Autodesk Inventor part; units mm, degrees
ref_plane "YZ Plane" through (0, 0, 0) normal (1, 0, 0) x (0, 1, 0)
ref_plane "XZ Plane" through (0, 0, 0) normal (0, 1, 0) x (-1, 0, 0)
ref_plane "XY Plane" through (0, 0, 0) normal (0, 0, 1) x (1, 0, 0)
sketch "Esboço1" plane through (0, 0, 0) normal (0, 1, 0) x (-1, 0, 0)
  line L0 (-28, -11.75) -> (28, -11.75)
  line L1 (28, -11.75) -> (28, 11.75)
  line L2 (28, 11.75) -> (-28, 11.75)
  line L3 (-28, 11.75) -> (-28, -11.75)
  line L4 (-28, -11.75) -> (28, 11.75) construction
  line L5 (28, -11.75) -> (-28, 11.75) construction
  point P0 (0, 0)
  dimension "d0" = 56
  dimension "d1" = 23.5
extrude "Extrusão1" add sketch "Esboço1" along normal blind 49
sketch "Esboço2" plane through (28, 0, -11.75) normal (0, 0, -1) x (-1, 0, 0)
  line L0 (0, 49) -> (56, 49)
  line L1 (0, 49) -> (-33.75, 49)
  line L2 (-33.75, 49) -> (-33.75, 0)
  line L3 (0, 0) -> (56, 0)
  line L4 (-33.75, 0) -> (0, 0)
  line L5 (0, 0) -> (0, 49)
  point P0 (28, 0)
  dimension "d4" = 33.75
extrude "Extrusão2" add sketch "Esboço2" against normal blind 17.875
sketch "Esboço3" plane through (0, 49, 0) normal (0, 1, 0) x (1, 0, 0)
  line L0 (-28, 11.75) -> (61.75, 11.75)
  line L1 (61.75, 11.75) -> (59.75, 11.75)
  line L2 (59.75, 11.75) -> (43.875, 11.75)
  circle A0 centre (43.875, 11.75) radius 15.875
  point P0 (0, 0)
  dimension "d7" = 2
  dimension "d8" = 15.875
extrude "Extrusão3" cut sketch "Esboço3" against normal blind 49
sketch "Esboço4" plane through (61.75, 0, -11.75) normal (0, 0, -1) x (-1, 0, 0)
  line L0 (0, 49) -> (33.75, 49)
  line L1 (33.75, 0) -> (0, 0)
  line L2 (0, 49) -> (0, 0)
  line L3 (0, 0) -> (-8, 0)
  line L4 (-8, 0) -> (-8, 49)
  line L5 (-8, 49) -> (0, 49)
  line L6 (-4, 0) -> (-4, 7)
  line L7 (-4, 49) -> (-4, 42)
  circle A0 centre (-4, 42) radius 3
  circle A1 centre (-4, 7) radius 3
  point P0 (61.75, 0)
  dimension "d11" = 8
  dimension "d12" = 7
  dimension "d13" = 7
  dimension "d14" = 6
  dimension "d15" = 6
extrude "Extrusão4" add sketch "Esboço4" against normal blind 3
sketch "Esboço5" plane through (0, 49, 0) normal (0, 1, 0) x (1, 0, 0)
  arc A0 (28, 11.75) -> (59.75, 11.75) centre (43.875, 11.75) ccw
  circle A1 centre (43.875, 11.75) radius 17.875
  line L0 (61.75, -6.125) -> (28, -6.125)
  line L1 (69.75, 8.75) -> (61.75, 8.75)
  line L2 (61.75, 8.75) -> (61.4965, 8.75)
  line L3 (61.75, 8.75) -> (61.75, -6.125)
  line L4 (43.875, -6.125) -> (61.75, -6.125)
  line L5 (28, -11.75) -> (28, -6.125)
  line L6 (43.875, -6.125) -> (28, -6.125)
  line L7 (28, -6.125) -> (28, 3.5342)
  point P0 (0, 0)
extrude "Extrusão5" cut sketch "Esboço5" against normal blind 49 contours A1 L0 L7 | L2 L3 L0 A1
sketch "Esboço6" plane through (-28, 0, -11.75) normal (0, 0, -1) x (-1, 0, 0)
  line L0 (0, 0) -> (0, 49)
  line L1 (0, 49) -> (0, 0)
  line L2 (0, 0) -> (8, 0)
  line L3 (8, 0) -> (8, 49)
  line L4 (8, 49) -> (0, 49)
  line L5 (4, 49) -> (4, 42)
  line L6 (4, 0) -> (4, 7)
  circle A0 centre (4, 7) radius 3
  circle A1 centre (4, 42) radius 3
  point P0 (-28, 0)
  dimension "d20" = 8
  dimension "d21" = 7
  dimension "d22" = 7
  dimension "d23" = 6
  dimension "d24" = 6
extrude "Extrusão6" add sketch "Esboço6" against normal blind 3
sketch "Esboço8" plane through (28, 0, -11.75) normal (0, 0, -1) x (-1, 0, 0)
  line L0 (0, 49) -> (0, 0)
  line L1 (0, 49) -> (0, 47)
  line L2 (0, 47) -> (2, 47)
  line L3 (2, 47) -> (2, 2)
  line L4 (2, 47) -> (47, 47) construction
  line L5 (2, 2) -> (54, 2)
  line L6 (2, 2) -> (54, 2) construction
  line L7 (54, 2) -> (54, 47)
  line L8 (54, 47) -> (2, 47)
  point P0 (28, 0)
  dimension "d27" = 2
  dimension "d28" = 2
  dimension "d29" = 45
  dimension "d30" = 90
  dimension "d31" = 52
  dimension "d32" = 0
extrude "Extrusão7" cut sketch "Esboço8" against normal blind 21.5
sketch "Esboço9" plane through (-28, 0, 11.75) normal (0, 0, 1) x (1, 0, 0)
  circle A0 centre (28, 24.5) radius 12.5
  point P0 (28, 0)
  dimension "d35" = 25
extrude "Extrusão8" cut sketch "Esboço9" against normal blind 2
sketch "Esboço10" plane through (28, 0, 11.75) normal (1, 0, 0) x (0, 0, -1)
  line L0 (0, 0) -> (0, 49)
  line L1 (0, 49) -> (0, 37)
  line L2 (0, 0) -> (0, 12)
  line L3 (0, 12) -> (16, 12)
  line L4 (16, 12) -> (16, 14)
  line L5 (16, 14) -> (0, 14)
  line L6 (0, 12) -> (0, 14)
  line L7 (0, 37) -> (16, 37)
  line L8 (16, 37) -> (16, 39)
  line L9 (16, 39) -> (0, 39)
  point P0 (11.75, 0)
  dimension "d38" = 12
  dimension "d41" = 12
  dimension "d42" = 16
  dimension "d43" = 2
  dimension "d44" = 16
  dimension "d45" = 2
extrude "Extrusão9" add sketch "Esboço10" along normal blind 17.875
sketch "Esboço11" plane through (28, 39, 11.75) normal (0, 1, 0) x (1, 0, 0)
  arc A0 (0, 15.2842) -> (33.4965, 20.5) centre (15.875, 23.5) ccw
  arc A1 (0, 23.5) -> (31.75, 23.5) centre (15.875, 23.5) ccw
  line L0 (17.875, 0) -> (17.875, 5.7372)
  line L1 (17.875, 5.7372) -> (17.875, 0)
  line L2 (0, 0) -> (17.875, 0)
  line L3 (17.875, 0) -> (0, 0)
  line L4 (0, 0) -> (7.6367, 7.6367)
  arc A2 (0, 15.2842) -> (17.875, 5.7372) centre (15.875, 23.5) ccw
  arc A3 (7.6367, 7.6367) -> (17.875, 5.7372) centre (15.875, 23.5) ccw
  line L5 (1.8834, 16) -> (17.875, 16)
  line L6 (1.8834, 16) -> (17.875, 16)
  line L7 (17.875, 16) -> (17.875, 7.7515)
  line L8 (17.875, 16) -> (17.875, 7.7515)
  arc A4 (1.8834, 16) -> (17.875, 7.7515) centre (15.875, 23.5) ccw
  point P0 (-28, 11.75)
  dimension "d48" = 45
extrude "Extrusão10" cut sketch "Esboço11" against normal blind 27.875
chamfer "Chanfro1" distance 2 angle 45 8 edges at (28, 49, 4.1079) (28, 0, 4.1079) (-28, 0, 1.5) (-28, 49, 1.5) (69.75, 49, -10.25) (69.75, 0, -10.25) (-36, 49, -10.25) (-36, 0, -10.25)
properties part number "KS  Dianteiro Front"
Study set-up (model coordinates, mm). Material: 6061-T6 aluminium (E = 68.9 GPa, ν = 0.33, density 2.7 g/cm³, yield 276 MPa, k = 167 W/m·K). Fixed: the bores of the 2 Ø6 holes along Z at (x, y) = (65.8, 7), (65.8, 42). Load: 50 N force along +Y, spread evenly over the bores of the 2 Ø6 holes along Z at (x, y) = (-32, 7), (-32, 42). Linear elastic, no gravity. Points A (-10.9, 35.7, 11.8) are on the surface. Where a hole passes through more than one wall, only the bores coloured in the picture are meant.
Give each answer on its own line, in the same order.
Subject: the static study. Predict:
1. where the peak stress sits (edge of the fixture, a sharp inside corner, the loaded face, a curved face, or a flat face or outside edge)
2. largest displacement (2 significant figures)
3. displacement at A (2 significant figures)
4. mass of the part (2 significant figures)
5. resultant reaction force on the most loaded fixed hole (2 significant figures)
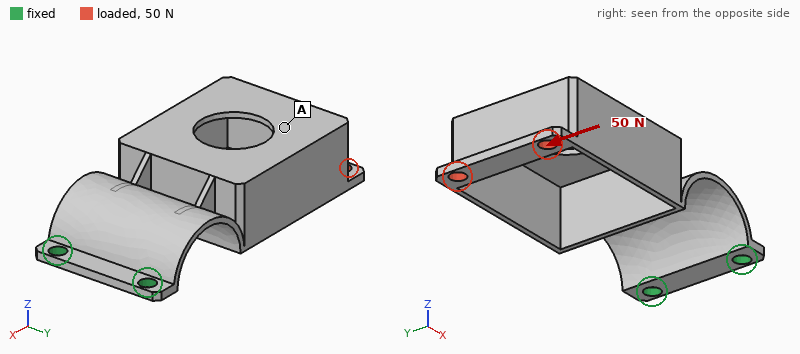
a curved face
0.78 mm
0.31 mm
54 g
130 N
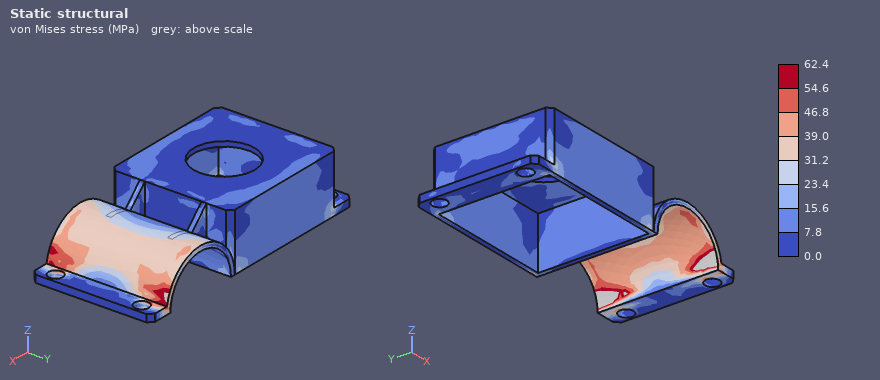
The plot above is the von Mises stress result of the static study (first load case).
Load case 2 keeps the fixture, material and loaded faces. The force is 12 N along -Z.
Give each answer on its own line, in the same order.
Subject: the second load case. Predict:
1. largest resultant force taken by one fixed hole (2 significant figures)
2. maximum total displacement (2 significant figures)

22 N
1.3 mm
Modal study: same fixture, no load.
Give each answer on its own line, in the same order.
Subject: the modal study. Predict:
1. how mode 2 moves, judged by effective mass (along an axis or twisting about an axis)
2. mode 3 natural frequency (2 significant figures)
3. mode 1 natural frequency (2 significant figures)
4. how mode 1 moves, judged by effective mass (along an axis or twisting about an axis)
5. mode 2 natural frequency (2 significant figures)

along Y
840 Hz
120 Hz
along Z
340 Hz
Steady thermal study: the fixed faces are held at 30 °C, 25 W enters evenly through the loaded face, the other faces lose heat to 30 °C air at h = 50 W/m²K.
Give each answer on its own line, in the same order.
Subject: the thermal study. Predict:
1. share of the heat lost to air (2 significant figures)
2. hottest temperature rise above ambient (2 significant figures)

84 %
64 K
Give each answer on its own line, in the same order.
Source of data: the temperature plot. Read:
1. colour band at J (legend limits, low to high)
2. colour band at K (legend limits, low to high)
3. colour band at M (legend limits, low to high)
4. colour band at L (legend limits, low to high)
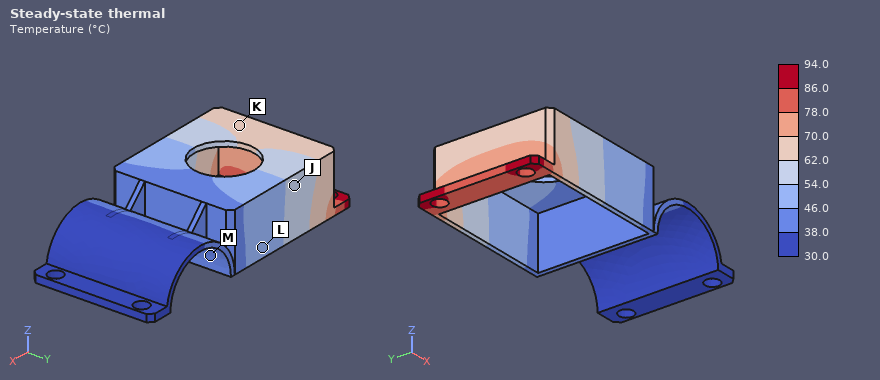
54.0 to 62.0 °C
62.0 to 70.0 °C
38.0 to 46.0 °C
46.0 to 54.0 °C
